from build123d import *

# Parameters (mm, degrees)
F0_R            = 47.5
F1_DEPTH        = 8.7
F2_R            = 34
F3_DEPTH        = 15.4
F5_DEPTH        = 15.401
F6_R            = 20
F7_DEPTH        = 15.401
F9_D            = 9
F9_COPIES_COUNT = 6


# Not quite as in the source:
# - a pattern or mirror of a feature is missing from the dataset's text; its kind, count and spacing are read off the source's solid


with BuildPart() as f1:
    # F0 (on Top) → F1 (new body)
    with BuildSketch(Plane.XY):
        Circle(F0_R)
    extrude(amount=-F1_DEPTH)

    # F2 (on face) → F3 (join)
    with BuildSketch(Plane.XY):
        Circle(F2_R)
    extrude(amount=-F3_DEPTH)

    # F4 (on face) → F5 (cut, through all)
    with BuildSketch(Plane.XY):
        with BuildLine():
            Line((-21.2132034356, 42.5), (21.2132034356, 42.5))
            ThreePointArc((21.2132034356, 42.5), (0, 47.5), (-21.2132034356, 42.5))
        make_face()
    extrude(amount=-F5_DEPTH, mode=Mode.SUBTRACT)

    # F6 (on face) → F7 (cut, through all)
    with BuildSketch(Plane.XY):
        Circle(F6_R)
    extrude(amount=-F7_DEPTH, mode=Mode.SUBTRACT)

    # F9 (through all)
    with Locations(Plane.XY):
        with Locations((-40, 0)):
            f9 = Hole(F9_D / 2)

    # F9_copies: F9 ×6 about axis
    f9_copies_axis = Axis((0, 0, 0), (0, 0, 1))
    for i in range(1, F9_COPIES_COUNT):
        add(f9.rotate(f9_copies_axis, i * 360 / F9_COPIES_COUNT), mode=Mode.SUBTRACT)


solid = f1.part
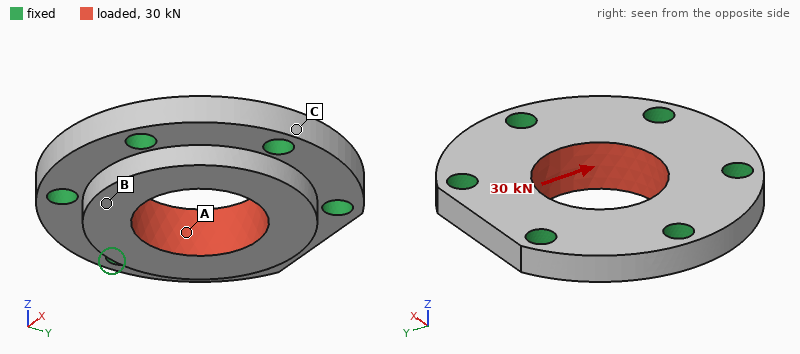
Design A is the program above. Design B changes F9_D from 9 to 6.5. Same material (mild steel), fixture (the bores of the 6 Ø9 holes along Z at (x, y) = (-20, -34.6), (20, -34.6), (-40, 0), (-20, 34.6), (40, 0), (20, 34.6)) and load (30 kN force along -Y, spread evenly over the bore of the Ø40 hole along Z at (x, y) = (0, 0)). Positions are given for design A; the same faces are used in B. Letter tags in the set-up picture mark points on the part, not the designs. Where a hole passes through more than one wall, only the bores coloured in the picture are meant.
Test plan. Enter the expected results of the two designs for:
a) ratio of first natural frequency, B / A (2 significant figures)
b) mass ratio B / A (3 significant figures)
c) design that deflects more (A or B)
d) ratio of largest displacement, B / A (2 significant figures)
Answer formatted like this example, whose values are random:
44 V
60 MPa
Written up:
0.88
1.03
B
1.1
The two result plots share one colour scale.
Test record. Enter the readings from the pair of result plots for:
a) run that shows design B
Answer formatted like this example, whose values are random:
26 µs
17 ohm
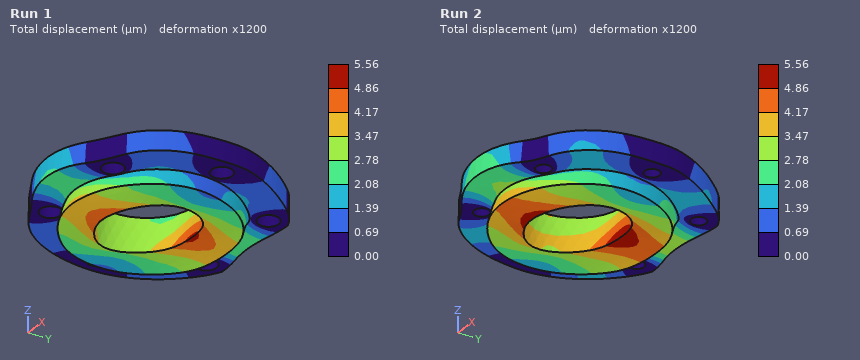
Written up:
Run 2
